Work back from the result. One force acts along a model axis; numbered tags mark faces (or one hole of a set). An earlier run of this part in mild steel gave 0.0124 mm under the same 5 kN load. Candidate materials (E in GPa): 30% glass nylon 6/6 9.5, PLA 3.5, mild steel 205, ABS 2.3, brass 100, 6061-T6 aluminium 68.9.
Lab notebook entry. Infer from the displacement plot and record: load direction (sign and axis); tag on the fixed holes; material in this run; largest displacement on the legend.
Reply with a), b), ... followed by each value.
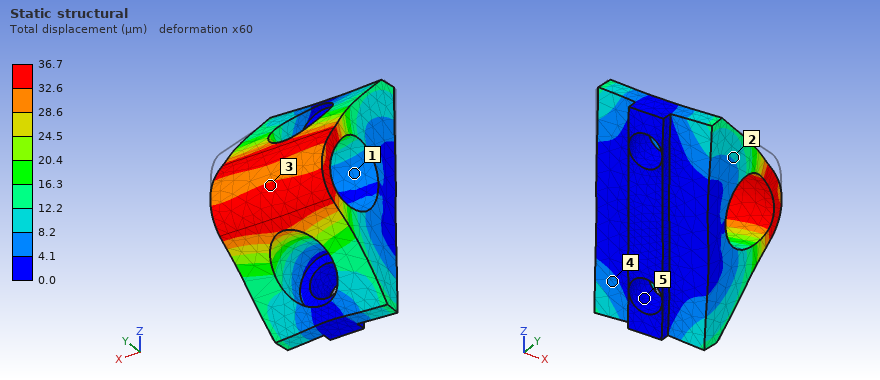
a) -Z
b) 5
c) 6061-T6 aluminium
d) 36.7 µm
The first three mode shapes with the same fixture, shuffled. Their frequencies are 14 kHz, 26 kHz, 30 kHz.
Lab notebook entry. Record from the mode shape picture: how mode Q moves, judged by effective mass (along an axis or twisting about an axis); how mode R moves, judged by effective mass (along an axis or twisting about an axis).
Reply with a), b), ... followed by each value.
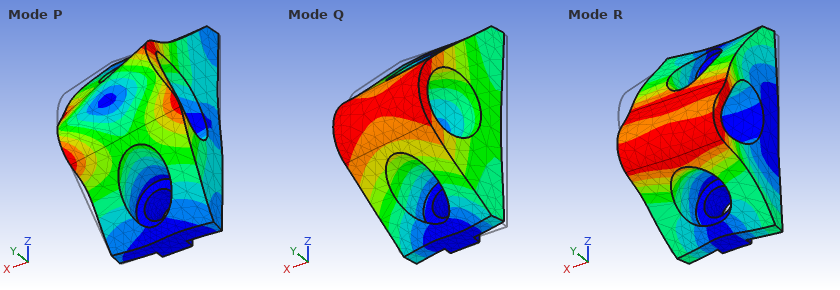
a) along X
b) along Z
